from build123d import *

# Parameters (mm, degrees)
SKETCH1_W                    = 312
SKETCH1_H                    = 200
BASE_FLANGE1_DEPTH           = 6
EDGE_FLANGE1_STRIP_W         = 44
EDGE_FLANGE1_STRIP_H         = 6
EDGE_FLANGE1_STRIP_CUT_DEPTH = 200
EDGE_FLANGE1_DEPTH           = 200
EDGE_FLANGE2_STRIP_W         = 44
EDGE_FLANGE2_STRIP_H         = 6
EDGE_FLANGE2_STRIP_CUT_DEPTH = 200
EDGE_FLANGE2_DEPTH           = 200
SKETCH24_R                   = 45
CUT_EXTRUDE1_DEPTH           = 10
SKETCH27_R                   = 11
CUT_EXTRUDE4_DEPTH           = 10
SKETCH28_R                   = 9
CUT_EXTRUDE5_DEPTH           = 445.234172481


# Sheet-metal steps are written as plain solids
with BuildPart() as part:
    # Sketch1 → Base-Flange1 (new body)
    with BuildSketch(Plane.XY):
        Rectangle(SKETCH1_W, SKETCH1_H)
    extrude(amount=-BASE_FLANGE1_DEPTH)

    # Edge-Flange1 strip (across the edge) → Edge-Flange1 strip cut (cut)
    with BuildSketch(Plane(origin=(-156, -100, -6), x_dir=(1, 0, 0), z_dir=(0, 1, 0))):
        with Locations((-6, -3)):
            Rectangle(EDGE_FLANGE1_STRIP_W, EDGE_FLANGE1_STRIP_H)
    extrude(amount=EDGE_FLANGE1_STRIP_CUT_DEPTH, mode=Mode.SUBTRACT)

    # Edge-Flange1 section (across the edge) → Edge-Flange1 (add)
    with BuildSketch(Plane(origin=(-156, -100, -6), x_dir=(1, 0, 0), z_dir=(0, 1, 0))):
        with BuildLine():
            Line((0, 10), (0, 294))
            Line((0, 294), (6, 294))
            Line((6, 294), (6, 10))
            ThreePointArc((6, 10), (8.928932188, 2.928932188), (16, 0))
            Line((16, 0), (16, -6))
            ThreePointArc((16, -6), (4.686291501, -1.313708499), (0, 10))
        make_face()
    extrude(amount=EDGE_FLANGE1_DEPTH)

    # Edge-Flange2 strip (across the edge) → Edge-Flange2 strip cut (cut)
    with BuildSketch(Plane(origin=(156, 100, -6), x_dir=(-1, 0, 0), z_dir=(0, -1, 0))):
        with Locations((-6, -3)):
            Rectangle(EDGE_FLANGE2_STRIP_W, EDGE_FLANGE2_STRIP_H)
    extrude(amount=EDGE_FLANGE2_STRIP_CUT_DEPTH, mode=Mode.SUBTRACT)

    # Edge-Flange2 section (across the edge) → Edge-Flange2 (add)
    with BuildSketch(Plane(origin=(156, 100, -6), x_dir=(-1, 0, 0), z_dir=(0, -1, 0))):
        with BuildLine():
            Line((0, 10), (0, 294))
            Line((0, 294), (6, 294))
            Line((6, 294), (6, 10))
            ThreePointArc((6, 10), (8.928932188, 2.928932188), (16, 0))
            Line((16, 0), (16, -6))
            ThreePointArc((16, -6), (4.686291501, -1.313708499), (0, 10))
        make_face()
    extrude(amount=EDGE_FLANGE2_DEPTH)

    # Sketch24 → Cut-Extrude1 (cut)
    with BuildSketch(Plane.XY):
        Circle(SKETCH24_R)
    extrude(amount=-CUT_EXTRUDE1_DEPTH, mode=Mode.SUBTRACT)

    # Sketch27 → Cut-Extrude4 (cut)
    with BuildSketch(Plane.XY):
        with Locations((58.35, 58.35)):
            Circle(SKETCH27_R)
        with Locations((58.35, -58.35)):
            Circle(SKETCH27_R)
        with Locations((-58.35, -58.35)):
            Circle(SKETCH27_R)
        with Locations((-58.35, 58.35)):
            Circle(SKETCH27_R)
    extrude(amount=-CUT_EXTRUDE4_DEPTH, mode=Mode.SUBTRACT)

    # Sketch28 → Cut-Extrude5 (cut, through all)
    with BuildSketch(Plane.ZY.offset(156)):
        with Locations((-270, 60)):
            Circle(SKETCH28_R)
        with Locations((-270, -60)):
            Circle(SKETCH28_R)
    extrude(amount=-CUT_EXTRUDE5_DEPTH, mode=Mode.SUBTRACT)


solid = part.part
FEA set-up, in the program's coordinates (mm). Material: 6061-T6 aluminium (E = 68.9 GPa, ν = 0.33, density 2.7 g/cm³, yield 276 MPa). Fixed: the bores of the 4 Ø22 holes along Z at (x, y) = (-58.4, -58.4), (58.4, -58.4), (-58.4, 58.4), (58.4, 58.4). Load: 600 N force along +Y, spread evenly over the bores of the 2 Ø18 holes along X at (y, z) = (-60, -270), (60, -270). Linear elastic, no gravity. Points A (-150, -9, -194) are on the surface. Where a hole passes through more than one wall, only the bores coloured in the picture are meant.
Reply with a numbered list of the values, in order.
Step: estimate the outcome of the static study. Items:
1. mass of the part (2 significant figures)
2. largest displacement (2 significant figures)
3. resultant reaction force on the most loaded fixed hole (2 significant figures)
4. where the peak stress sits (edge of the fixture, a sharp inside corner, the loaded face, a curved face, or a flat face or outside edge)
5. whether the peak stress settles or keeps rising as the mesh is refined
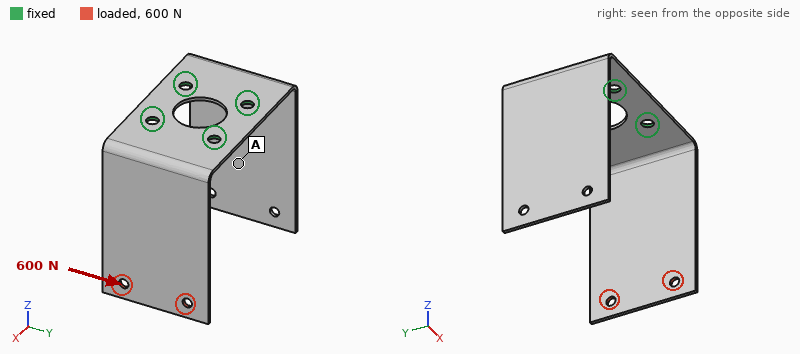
1. 2.7 kg
2. 4.5 mm
3. 1.3 kN
4. edge of the fixture
5. keeps rising
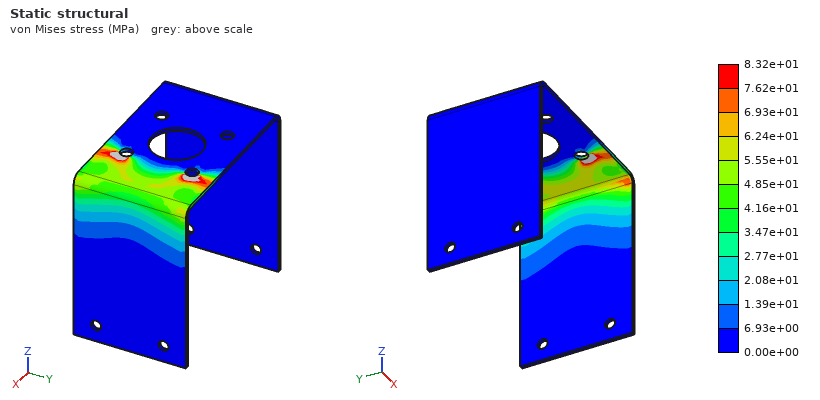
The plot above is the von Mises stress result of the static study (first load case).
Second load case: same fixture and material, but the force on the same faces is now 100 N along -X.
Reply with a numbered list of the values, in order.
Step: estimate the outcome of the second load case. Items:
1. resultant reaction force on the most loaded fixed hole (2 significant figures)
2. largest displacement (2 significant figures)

1. 66 N
2. 5.3 mm
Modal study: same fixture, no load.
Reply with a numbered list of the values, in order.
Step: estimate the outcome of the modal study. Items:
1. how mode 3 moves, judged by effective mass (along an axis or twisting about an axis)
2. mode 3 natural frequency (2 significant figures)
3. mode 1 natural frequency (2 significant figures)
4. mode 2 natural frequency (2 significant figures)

1. along Y
2. 94 Hz
3. 39 Hz
4. 39 Hz
